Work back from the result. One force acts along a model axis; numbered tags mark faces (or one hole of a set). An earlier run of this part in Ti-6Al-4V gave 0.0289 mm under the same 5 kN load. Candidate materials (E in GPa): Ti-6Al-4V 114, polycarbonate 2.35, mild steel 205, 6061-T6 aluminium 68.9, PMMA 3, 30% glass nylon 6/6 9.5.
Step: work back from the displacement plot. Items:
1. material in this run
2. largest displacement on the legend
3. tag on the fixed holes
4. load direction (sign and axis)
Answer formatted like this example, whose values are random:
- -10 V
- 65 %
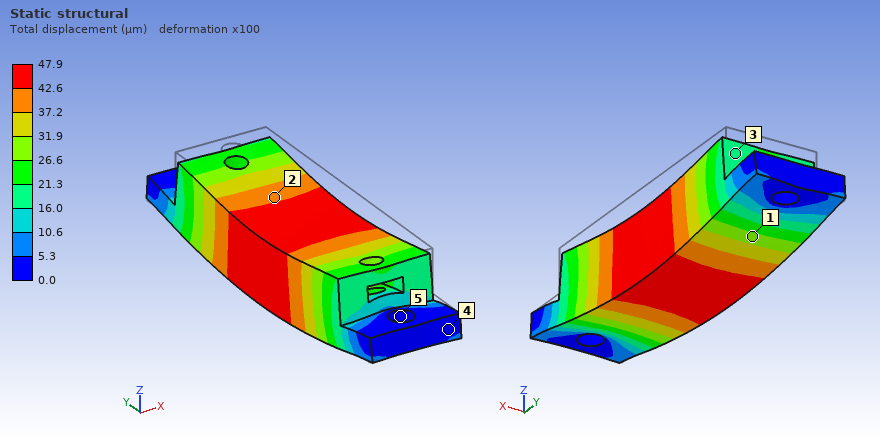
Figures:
- 6061-T6 aluminium
- 47.9 µm
- 5
- -Z
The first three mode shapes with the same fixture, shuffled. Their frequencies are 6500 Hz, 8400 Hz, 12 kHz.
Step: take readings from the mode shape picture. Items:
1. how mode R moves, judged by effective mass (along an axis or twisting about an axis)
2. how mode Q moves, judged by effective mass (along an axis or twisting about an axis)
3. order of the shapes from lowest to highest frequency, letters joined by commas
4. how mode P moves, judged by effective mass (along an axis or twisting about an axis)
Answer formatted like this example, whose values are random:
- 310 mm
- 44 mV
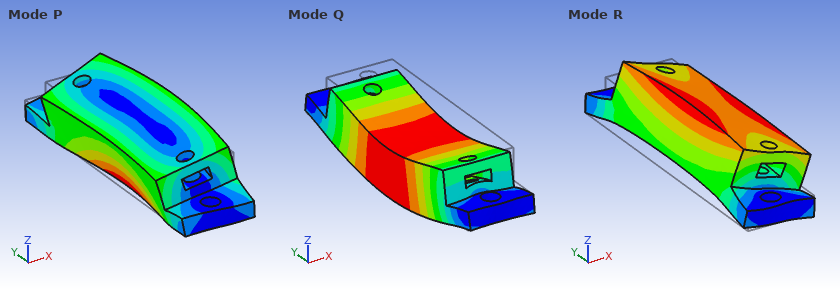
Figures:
- along X
- along Z
- R, Q, P
- along X
